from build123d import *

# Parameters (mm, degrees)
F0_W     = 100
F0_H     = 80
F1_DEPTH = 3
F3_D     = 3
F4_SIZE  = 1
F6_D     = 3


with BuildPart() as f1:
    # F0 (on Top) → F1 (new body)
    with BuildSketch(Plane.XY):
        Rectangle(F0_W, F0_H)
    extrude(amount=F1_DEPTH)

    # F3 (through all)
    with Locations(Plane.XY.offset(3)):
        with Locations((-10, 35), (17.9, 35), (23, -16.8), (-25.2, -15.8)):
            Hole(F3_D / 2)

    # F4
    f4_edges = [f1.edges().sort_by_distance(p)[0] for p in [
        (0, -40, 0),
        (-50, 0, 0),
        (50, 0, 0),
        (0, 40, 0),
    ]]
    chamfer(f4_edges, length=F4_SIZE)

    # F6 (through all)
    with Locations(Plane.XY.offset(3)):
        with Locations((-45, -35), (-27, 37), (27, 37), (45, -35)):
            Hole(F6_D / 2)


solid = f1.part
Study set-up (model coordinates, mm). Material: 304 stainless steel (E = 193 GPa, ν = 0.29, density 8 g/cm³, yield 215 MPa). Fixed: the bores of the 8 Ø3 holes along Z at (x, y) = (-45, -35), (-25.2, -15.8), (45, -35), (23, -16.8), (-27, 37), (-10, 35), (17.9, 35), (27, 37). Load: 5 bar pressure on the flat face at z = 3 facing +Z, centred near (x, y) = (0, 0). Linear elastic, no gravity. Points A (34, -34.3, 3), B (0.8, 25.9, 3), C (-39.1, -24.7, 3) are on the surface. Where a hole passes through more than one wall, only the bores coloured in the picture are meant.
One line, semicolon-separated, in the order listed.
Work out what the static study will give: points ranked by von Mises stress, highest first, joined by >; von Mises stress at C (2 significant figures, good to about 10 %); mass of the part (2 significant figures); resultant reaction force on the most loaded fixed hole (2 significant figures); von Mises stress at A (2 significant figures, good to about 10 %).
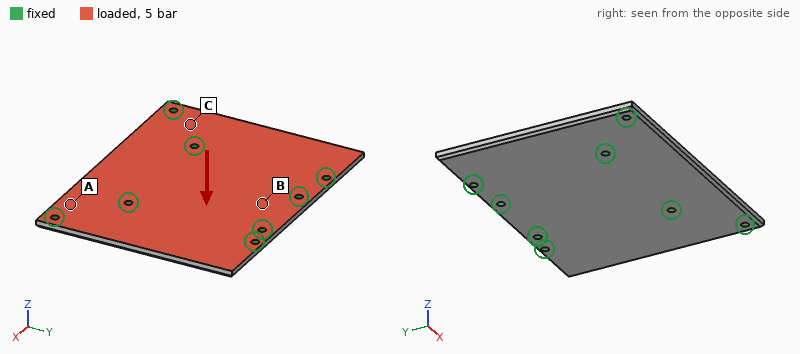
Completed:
C > A > B; 54 MPa; 190 g; 1.0 kN; 31 MPa
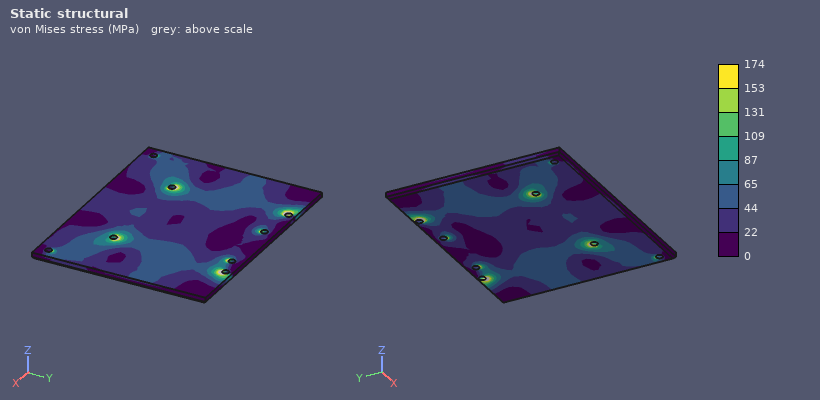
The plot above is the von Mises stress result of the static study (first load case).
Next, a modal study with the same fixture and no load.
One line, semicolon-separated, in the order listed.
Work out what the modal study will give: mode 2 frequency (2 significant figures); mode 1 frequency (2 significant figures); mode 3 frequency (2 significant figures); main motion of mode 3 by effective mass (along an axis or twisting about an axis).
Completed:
3200 Hz; 3100 Hz; 4000 Hz; along Z
